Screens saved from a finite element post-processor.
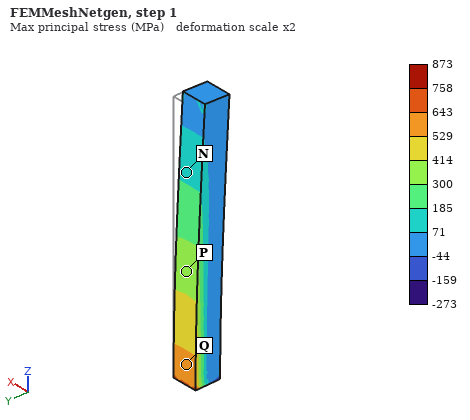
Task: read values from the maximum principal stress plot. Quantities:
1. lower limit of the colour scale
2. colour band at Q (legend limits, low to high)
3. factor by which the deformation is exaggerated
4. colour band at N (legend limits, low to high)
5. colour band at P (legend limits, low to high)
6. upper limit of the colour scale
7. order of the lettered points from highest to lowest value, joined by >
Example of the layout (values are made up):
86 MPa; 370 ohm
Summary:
-273 MPa; 529 to 643 MPa; 2; 71 to 185 MPa; 300 to 414 MPa; 873 MPa; Q > P > N
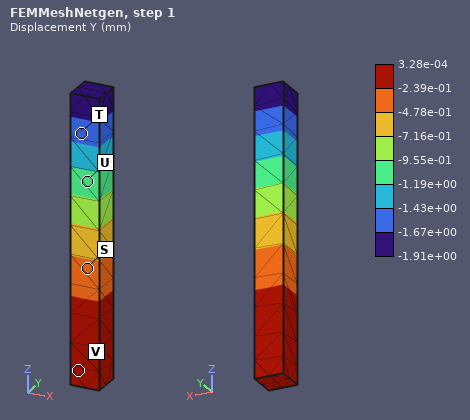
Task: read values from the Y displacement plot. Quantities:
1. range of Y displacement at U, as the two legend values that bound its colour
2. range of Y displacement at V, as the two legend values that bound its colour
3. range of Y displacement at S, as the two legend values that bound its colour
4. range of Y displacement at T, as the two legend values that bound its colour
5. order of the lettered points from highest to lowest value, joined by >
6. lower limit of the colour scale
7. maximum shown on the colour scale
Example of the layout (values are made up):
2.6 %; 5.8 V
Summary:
-1.19e+00 to -9.55e-01 mm; -2.39e-01 to 3.28e-04 mm; -4.78e-01 to -2.39e-01 mm; -1.67e+00 to -1.43e+00 mm; V > S > U > T; -1.91e+00 mm; 3.28e-04 mm
